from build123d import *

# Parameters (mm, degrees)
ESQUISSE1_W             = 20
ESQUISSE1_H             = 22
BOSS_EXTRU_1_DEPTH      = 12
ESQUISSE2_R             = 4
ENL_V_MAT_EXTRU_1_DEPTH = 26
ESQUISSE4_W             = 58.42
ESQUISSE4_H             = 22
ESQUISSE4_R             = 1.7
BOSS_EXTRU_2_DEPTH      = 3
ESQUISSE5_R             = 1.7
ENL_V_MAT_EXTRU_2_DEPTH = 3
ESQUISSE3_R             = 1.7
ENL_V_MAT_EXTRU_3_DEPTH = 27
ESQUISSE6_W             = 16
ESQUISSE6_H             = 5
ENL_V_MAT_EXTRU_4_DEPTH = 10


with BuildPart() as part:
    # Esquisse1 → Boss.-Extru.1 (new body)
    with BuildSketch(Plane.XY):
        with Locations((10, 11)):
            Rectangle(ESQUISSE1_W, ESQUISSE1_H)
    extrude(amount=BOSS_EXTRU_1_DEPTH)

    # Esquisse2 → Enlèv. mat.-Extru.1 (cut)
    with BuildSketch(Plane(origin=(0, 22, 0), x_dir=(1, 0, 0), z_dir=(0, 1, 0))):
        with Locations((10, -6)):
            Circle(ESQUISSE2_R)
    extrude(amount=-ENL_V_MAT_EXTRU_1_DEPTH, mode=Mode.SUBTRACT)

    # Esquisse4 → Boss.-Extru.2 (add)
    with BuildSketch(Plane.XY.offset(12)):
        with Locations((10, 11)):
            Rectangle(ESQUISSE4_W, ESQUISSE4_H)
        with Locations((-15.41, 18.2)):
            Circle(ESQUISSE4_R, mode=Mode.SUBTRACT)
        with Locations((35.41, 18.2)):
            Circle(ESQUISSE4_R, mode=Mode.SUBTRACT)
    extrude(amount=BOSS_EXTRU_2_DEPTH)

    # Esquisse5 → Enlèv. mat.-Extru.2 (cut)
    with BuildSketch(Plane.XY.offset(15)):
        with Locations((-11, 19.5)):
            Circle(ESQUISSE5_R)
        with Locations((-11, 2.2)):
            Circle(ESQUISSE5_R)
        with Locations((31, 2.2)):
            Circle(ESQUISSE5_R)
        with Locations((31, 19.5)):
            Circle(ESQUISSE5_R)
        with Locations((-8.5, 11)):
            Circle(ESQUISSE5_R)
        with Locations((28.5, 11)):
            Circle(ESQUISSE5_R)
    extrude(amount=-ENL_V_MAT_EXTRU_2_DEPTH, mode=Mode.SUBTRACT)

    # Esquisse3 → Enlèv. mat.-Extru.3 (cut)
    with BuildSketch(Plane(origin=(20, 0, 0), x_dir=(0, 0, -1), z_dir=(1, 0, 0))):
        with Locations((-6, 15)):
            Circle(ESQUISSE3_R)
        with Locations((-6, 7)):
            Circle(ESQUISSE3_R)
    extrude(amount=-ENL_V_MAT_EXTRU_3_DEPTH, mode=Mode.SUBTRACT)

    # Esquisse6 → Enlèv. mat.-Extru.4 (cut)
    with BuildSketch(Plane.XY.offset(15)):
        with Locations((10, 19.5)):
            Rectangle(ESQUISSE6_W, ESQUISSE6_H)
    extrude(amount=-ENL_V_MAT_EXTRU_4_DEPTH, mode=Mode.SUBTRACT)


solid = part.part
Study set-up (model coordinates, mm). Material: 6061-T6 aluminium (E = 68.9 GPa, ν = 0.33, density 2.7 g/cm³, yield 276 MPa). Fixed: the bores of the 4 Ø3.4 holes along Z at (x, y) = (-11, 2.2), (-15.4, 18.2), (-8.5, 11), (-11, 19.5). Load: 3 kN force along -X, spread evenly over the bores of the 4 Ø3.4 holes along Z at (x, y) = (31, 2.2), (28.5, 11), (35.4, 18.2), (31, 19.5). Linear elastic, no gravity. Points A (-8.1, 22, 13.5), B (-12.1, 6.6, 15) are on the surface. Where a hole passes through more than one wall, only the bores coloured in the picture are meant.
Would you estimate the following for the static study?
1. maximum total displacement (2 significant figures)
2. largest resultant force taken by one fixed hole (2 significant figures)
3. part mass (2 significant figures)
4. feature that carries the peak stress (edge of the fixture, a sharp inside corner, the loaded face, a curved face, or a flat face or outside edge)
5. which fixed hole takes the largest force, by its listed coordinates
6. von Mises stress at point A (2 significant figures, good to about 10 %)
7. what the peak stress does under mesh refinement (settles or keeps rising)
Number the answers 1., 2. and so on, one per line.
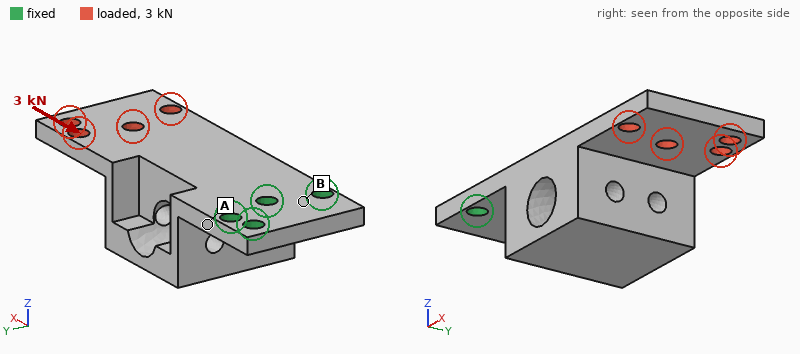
1. 0.15 mm
2. 1.5 kN
3. 19 g
4. a sharp inside corner
5. (-8.5, 11)
6. 44 MPa
7. keeps rising
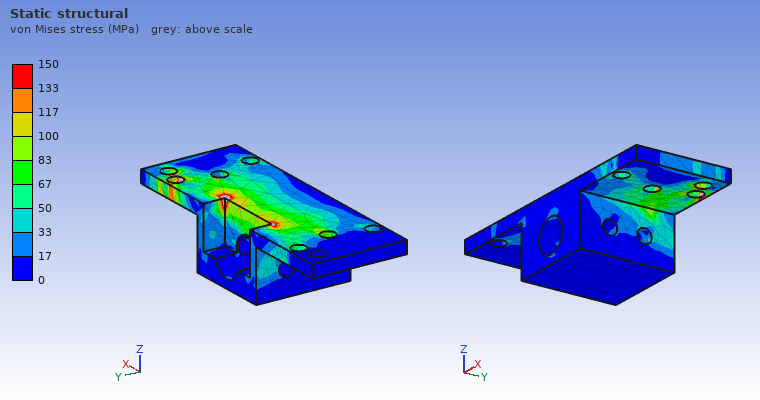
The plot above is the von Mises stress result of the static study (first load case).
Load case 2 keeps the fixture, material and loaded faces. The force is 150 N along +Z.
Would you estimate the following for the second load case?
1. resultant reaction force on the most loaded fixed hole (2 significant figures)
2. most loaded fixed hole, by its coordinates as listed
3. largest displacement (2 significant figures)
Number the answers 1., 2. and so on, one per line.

1. 380 N
2. (-8.5, 11)
3. 0.74 mm
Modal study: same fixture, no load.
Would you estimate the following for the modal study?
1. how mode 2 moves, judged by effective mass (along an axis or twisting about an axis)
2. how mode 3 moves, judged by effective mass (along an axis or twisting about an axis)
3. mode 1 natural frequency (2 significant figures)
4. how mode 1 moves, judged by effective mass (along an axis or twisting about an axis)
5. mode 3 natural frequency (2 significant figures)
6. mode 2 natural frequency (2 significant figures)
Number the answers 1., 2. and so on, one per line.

1. along Y
2. along Y
3. 1100 Hz
4. along Z
5. 5600 Hz
6. 4600 Hz
